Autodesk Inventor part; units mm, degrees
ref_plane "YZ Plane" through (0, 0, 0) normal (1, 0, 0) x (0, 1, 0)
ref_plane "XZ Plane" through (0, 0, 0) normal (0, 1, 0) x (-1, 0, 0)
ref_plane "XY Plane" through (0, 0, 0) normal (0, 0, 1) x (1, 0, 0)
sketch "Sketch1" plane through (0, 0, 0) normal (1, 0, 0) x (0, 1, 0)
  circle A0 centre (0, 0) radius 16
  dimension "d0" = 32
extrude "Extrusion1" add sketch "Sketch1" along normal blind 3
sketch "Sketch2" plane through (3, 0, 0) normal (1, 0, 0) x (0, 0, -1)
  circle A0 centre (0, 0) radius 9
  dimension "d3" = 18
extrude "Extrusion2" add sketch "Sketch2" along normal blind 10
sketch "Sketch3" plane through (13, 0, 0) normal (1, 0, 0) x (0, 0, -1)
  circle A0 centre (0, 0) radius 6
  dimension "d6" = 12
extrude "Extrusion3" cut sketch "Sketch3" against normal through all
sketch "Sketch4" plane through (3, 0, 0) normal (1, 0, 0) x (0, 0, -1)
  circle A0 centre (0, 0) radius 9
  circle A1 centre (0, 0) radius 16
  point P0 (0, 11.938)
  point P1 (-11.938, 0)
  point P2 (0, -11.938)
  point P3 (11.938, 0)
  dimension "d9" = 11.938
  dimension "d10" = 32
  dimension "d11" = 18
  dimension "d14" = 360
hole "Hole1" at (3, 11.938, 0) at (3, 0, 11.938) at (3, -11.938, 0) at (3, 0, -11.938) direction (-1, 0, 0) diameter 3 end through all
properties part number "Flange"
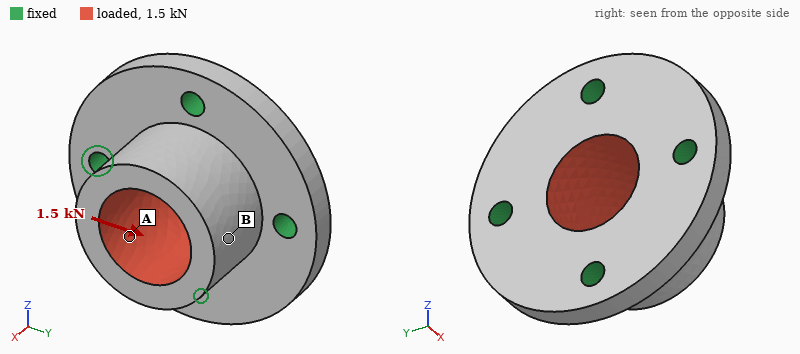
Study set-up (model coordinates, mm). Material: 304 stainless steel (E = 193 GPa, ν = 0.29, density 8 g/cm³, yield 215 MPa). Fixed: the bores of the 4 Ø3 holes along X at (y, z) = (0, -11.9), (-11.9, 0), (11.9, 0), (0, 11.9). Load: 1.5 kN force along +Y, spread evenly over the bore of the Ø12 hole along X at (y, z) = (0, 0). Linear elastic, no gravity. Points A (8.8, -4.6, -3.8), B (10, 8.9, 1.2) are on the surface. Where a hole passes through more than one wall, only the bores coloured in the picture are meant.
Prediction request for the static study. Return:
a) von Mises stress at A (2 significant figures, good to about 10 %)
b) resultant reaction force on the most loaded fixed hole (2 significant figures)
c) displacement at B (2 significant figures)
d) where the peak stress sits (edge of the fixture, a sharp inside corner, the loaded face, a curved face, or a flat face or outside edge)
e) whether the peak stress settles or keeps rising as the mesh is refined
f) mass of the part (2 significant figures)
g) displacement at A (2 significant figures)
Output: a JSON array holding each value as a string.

["14 MPa", "540 N", "2.5 µm", "edge of the fixture", "keeps rising", "27 g", "2.1 µm"]
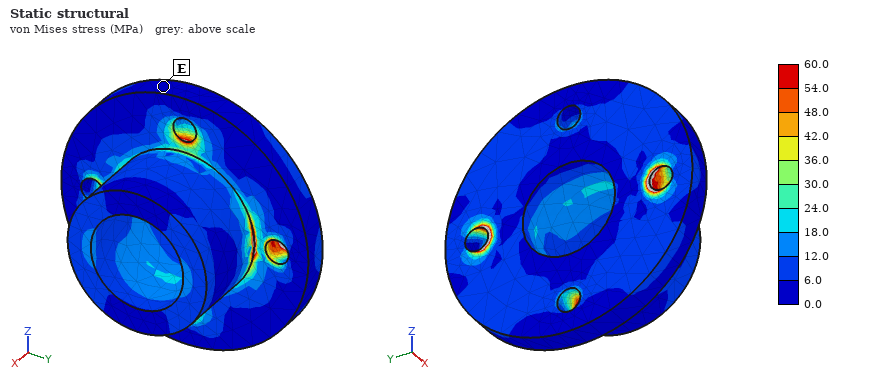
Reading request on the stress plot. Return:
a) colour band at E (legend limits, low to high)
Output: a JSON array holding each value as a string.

["0.0 to 6.0 MPa"]
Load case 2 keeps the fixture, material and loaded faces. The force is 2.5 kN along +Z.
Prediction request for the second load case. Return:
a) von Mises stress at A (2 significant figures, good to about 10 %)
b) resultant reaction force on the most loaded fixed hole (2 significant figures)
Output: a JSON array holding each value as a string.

["24 MPa", "910 N"]
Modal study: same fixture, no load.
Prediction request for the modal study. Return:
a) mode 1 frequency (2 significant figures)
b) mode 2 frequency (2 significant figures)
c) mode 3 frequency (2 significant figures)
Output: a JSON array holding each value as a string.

["31 kHz", "31 kHz", "35 kHz"]
